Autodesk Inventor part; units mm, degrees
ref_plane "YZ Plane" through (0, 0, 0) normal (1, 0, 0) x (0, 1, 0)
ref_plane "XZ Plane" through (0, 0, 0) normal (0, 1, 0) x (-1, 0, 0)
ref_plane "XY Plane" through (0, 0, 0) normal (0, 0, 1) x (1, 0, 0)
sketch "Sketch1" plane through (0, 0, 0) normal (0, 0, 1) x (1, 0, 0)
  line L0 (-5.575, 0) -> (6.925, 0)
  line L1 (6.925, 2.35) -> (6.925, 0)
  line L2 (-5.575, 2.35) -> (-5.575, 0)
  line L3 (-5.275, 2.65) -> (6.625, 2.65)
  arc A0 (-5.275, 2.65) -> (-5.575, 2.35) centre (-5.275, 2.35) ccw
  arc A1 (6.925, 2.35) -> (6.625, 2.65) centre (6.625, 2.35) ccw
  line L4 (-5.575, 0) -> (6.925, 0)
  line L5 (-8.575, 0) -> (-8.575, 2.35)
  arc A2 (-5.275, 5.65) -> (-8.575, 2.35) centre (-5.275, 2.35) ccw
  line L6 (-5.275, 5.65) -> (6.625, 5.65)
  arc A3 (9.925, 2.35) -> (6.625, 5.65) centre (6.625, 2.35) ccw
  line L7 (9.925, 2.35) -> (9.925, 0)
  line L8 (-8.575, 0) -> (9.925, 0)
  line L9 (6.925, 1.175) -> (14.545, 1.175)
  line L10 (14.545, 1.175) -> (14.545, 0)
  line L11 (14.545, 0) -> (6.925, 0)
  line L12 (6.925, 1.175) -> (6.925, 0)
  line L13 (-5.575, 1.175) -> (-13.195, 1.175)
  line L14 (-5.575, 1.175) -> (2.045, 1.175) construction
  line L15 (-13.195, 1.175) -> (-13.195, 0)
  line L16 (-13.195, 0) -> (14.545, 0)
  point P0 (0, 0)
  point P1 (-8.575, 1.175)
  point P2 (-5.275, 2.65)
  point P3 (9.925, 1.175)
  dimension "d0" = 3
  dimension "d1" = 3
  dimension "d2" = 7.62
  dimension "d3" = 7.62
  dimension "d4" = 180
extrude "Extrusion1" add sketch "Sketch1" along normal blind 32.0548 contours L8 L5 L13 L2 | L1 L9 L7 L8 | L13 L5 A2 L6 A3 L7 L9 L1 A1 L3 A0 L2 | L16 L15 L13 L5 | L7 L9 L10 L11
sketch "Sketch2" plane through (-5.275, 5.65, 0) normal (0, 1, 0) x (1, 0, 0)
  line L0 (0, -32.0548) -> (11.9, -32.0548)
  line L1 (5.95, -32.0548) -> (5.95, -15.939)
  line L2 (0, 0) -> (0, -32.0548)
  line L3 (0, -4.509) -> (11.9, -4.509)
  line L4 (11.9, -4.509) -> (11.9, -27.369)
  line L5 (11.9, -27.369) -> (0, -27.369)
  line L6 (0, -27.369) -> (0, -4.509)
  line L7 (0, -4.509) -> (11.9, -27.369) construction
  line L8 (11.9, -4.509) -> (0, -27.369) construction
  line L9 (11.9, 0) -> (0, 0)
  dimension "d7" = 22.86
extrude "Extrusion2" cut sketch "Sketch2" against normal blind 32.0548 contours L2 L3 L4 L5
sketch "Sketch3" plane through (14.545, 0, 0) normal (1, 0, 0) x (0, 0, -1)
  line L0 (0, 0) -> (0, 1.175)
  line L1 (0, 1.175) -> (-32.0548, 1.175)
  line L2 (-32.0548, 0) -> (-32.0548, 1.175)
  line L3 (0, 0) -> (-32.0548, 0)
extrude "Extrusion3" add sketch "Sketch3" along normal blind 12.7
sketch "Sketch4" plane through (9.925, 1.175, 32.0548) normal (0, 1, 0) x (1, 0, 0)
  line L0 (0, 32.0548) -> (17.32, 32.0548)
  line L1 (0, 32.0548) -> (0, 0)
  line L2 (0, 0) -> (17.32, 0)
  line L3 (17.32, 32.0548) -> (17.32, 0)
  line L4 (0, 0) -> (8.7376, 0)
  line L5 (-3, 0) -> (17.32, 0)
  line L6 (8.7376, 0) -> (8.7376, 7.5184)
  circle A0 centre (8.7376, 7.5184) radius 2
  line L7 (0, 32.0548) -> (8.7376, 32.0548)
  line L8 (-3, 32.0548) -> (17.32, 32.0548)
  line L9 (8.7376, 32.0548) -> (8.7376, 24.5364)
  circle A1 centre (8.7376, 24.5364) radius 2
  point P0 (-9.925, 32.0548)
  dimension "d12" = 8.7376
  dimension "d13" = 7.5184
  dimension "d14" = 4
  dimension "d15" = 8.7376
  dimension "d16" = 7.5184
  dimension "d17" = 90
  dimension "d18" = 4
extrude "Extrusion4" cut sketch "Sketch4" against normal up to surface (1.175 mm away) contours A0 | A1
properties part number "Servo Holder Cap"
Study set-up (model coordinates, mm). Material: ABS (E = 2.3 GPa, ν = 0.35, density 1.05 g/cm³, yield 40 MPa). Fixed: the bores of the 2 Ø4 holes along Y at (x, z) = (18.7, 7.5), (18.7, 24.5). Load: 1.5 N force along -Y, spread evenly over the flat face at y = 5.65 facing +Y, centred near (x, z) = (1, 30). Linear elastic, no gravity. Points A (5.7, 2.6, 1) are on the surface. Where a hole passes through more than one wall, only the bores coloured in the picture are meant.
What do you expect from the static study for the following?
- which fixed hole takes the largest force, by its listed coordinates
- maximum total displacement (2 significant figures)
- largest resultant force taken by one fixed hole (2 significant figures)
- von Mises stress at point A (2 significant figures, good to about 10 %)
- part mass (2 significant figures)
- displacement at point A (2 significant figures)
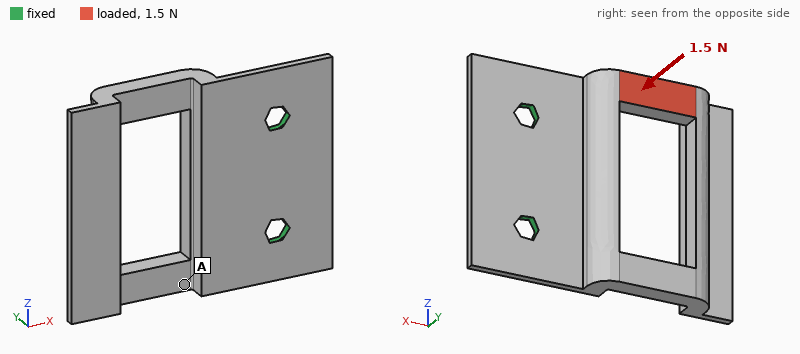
(18.7, 24.5)
0.50 mm
1.7 N
0.73 MPa
2.2 g
0.093 mm
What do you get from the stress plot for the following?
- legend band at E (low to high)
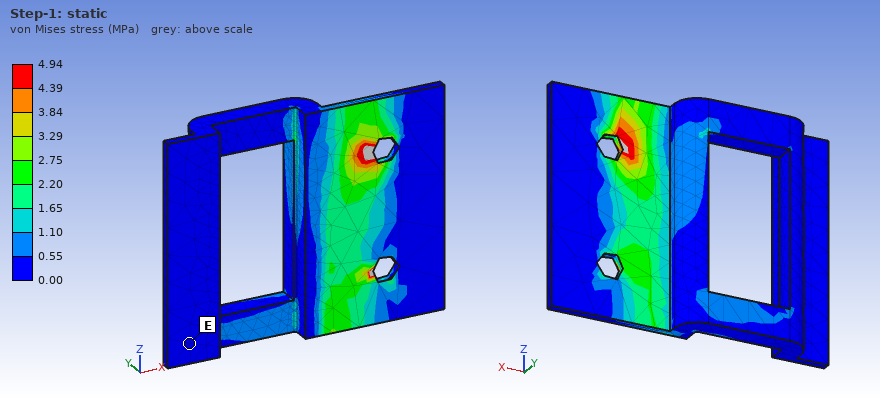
0.00 to 0.55 MPa
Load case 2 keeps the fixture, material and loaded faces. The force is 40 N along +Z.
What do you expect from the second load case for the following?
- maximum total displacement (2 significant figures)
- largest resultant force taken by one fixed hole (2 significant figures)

0.40 mm
42 N
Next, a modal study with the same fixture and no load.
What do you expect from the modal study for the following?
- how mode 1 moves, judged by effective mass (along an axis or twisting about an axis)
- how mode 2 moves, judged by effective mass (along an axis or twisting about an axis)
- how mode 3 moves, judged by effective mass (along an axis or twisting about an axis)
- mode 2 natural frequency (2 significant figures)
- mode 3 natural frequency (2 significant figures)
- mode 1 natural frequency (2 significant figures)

along Y
twisting about X
along Z
910 Hz
1700 Hz
270 Hz
